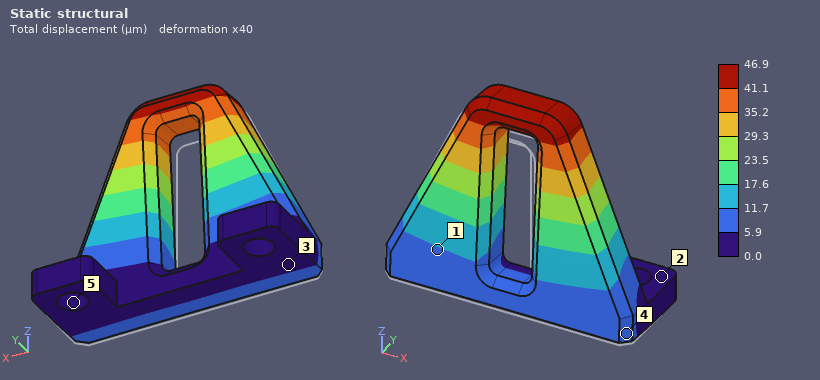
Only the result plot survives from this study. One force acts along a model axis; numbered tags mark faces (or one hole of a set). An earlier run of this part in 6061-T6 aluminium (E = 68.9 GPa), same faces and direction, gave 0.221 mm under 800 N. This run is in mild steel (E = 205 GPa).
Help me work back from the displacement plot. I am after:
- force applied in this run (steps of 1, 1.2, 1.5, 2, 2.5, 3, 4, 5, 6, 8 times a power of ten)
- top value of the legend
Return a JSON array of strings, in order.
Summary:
["500 N", "46.9 µm"]
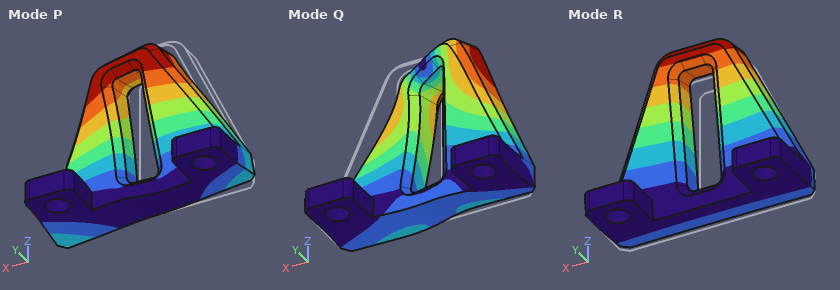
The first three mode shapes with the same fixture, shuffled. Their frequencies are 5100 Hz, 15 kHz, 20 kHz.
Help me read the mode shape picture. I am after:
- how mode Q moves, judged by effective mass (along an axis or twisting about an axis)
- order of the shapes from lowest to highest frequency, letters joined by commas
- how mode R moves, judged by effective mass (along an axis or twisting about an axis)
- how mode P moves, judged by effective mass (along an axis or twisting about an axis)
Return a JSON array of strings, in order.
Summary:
["along X", "R, P, Q", "along Y", "along X"]
